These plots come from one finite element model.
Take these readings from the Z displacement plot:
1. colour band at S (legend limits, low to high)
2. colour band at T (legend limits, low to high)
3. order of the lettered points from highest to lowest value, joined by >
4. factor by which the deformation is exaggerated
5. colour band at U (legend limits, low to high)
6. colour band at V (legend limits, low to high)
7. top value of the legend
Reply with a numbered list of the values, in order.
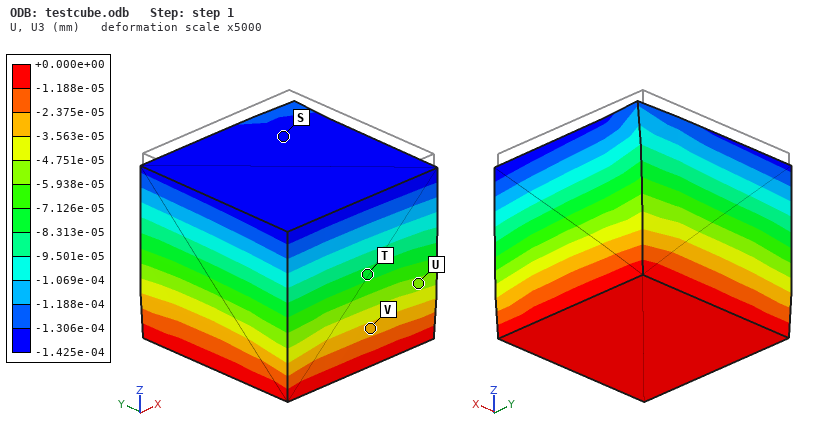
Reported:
1. -1.425e-04 to -1.306e-04 mm
2. -8.313e-05 to -7.126e-05 mm
3. V > U > T > S
4. 5000
5. -5.938e-05 to -4.751e-05 mm
6. -3.563e-05 to -2.375e-05 mm
7. +0.000e+00 mm
